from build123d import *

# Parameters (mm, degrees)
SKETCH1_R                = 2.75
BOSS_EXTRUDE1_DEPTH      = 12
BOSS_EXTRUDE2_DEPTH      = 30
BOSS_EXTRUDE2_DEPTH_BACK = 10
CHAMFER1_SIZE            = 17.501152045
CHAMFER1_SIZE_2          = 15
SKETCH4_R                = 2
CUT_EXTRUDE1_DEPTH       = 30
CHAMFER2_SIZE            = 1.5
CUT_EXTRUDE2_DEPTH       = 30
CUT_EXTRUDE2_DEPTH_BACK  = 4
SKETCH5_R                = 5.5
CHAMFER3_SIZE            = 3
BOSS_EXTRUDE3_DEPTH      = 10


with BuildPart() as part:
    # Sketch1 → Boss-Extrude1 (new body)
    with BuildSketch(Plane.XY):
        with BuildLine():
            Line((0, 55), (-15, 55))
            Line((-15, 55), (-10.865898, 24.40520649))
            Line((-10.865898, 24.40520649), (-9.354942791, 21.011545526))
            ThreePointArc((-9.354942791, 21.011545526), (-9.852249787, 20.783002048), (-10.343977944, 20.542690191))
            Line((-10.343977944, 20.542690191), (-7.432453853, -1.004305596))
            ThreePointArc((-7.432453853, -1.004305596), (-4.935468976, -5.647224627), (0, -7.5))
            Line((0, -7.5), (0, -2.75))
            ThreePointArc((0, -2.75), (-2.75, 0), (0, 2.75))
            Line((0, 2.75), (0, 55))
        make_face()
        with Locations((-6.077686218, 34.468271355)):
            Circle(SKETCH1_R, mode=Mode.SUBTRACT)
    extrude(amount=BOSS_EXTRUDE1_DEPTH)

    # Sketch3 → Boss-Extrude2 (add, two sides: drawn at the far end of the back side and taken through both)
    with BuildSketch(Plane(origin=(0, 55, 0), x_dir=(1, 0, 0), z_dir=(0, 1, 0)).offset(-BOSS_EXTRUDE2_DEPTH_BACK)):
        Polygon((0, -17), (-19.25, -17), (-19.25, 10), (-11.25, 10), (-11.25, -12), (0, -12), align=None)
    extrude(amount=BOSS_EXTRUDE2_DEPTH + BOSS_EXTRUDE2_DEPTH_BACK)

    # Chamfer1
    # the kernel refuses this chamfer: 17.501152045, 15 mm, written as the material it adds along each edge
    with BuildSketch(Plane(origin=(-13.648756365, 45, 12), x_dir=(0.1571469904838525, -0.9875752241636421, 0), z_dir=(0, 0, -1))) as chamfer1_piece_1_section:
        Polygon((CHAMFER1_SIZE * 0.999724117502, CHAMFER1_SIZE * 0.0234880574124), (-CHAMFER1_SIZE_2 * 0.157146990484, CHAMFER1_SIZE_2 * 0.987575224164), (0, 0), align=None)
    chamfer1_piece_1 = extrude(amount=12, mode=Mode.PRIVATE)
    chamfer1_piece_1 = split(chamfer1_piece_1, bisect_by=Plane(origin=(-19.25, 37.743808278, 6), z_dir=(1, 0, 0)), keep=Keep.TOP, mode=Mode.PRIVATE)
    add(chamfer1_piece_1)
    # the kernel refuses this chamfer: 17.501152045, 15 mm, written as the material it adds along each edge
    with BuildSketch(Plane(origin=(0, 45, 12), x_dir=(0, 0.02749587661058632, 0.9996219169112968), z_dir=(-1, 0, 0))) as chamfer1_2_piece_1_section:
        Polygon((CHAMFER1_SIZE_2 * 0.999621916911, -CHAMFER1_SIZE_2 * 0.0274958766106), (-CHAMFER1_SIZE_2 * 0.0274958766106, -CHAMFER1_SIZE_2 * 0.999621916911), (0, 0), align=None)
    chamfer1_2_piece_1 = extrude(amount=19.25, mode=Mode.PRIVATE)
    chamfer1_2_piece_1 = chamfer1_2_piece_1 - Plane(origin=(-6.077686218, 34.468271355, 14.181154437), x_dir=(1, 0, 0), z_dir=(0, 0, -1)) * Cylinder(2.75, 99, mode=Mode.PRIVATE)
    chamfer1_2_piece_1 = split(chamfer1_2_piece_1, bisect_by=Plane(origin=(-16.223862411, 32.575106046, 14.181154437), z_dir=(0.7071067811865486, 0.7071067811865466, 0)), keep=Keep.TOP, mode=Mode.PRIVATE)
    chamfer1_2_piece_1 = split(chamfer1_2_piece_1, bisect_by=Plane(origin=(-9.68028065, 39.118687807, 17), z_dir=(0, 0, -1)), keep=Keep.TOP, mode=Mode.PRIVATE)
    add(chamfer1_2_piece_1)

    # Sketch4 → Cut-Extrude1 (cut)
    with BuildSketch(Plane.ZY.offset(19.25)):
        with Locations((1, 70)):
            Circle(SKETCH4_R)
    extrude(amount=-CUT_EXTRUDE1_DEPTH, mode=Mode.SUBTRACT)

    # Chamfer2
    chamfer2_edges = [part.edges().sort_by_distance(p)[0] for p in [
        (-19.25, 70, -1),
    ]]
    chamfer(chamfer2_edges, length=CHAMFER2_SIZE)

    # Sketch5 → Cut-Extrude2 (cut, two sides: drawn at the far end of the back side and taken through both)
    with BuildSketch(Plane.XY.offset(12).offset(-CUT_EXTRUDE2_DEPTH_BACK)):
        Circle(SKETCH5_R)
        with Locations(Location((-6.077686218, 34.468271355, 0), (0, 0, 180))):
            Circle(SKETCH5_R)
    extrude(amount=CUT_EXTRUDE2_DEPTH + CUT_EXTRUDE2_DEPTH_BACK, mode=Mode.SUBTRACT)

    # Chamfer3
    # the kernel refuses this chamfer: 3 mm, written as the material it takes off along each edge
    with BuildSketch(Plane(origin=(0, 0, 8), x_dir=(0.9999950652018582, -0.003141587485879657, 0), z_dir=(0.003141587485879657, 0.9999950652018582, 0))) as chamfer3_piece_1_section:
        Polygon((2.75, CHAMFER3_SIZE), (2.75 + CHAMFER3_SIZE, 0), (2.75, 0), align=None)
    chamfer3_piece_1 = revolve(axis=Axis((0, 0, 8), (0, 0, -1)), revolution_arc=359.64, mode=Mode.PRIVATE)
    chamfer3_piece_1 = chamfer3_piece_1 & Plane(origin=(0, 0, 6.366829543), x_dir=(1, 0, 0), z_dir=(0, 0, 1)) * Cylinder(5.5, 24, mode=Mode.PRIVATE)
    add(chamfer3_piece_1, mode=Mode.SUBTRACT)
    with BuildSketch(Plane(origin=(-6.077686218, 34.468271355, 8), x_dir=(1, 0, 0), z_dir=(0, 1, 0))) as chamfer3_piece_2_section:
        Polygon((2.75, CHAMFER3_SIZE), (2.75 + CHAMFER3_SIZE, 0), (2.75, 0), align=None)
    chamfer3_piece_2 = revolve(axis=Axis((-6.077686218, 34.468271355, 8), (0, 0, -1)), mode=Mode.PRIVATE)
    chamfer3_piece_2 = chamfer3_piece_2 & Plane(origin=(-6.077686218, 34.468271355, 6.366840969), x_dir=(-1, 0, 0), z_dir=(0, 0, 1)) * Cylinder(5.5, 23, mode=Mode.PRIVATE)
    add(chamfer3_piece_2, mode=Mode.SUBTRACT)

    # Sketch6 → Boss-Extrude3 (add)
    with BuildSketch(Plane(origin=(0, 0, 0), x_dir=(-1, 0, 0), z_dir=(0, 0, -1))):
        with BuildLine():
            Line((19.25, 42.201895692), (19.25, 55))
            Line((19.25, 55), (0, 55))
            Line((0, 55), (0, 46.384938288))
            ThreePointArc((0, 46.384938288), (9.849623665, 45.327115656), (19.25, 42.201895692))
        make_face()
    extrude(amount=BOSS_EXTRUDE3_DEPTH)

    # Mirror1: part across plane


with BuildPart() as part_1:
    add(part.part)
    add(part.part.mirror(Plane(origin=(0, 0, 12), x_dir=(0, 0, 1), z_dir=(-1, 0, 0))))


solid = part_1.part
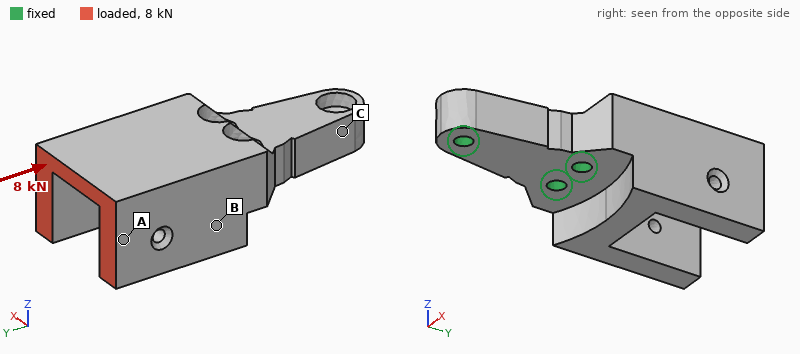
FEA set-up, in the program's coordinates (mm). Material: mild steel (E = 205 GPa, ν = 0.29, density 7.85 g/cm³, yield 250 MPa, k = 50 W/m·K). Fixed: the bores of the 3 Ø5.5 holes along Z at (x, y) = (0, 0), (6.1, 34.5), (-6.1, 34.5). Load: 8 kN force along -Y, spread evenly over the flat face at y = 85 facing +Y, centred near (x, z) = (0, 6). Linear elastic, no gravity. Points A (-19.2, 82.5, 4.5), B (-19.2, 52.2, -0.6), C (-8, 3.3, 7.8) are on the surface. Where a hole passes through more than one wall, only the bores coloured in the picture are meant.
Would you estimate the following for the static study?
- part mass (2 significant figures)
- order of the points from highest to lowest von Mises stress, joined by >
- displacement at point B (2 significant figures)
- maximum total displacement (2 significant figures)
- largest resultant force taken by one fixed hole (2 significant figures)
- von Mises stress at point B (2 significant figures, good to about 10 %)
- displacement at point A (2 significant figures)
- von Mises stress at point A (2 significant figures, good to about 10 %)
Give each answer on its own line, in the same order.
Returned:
320 g
B > A > C
4.6 µm
13 µm
3.5 kN
20 MPa
11 µm
14 MPa
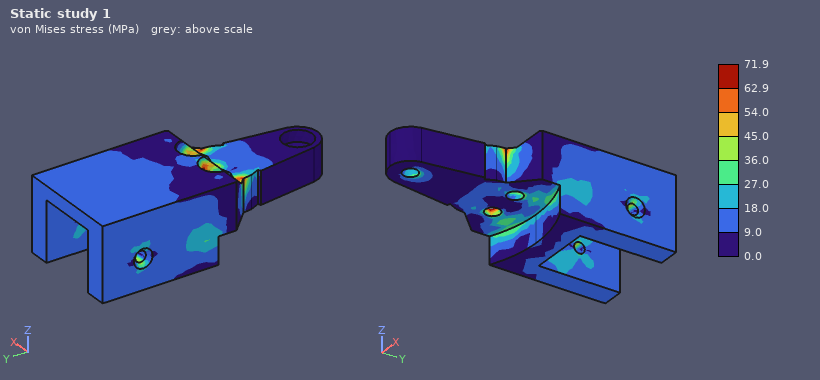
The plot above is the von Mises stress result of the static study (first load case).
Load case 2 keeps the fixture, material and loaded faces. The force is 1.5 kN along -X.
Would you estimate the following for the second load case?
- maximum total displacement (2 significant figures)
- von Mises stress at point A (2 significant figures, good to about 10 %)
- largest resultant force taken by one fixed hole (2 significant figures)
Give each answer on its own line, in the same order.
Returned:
32 µm
18 MPa
3.5 kN
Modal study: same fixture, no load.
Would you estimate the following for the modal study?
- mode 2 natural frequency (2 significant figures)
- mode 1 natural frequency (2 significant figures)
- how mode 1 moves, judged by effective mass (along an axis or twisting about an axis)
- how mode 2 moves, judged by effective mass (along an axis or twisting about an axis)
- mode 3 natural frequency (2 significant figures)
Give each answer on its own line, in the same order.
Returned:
4700 Hz
2700 Hz
along Z
along X
5900 Hz
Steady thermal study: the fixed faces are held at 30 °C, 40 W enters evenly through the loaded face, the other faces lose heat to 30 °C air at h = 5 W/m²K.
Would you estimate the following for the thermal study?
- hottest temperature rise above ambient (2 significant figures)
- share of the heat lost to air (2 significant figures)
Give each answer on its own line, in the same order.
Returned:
82 K
5.4 %
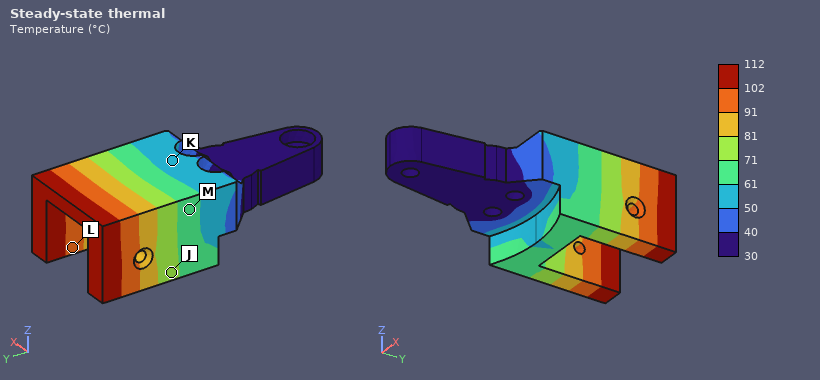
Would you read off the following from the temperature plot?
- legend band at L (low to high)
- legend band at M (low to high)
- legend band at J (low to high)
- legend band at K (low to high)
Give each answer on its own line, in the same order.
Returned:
91 to 102 °C
61 to 71 °C
71 to 81 °C
50 to 61 °C
